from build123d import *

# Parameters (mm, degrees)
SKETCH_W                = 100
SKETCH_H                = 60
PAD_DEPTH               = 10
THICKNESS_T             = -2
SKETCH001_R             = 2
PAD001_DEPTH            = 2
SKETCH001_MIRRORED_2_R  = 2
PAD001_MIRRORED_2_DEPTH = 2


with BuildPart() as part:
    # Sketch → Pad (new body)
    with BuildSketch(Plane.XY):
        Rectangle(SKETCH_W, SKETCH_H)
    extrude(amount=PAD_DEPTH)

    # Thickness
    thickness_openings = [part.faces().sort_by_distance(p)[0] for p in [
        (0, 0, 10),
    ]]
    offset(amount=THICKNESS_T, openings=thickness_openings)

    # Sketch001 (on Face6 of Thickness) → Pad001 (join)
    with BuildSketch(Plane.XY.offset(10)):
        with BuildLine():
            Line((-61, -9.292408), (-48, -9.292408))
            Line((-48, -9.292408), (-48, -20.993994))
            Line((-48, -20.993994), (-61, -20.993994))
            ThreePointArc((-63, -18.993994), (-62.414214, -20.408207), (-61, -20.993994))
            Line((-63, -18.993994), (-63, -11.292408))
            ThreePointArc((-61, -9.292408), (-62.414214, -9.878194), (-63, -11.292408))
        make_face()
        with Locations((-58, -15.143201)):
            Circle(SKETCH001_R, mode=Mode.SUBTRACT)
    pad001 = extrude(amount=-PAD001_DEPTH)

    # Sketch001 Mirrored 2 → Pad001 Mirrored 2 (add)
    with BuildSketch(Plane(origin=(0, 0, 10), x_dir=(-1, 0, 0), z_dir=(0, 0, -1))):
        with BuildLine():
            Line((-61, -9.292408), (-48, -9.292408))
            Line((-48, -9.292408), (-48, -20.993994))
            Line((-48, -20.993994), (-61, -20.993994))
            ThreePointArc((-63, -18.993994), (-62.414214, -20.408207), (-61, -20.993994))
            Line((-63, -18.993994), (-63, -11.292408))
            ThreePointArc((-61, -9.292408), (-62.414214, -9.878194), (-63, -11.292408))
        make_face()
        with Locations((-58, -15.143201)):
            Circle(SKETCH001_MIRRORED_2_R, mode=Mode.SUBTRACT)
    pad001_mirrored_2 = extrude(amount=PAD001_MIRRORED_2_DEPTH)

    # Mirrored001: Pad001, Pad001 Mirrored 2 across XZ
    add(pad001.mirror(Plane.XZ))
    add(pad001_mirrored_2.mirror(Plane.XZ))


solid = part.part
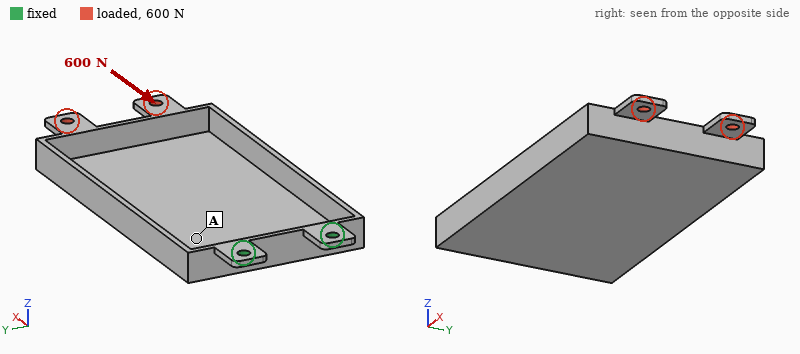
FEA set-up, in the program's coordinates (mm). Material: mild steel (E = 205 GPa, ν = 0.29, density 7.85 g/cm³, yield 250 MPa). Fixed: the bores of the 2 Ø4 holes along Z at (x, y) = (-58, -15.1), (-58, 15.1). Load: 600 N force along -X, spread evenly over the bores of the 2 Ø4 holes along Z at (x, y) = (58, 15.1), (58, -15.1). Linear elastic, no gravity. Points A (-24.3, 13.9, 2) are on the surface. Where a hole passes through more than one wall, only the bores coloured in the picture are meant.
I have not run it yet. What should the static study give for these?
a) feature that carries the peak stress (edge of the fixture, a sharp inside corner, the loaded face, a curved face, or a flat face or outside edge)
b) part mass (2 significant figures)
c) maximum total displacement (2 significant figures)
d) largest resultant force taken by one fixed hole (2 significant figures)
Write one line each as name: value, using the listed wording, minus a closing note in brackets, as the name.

feature that carries the peak stress: a flat face or outside edge
part mass: 140 g
maximum total displacement: 0.59 mm
largest resultant force taken by one fixed hole: 300 N
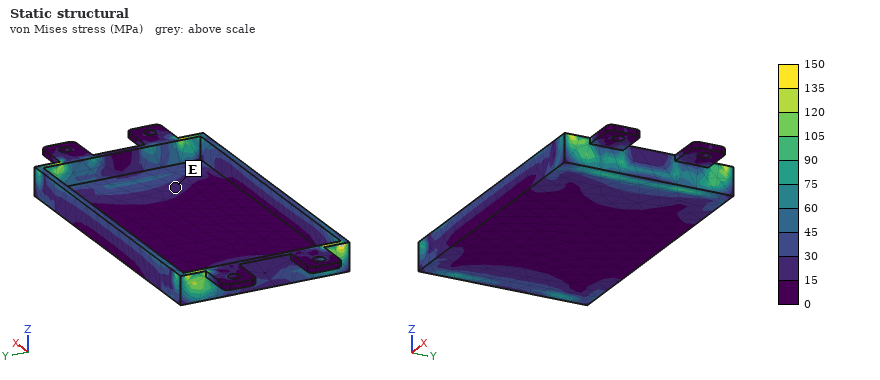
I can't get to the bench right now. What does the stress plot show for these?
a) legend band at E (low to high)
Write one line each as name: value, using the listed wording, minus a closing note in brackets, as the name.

legend band at E: 15 to 30 MPa
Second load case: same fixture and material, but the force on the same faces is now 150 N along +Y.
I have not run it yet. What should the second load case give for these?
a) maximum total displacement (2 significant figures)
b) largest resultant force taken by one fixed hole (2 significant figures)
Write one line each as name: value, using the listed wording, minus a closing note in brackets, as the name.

maximum total displacement: 0.49 mm
largest resultant force taken by one fixed hole: 440 N
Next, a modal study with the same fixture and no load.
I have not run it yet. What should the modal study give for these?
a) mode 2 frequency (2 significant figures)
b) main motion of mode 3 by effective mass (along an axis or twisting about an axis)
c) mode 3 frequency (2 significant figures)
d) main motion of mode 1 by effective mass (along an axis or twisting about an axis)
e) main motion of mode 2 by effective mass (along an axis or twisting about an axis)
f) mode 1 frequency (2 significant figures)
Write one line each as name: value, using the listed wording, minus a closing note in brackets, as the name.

mode 2 frequency: 410 Hz
main motion of mode 3 by effective mass: along Y
mode 3 frequency: 910 Hz
main motion of mode 1 by effective mass: along Z
main motion of mode 2 by effective mass: along Y
mode 1 frequency: 110 Hz
